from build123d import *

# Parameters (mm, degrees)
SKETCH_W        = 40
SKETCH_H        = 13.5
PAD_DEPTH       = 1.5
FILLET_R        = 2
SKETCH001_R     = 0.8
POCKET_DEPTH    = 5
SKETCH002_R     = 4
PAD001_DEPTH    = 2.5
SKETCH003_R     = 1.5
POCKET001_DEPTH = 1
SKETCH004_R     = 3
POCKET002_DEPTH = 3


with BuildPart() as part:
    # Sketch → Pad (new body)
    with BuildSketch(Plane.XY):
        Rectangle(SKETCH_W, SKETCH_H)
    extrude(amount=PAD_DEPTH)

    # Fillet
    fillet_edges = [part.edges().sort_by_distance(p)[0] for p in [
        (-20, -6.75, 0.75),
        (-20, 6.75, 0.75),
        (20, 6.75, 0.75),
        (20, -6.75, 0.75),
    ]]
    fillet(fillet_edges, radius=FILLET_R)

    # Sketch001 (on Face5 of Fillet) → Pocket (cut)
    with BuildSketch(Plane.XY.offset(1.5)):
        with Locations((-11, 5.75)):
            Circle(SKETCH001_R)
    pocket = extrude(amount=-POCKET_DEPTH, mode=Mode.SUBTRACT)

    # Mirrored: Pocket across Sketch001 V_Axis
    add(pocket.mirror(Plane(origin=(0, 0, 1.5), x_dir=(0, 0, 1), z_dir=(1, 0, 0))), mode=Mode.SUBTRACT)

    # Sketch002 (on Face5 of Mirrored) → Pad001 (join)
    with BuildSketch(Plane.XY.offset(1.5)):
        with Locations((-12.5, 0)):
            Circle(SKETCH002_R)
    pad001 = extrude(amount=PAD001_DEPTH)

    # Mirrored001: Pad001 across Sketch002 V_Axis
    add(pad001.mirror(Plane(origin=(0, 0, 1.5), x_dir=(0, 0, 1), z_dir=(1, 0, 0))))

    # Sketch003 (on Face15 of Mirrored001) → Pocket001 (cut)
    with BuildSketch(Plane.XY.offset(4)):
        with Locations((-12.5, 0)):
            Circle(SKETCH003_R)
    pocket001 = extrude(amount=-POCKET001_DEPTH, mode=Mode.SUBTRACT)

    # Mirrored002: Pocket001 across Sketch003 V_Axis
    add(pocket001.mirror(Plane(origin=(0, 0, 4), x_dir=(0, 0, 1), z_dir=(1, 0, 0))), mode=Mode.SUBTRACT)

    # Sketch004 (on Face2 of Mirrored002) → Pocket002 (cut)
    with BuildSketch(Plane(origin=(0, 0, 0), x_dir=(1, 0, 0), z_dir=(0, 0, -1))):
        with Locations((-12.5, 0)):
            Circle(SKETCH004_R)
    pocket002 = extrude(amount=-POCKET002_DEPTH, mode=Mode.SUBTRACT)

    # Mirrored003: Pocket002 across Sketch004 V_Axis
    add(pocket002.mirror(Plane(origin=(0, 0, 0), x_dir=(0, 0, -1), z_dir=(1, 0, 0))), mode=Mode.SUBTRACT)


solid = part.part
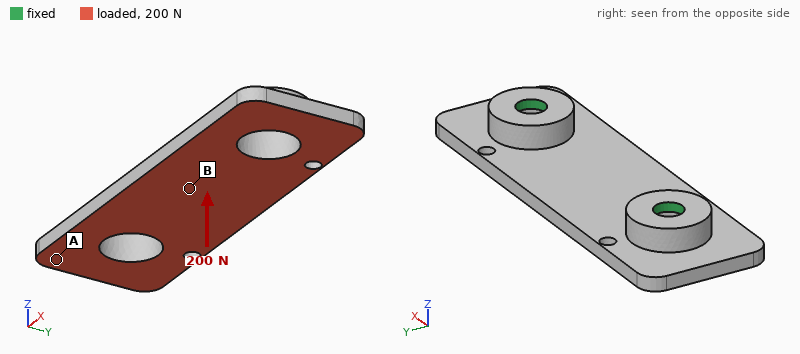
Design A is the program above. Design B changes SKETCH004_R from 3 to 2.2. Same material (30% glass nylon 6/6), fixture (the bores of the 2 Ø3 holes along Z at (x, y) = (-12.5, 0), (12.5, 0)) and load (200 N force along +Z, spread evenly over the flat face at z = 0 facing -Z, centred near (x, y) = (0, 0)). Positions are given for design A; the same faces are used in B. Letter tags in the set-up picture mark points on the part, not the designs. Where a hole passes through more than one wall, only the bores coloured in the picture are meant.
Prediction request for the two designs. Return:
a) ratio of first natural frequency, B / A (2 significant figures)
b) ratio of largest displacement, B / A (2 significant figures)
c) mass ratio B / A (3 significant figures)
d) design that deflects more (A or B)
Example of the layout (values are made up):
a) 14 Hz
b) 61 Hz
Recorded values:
a) 1.1
b) 0.82
c) 1.09
d) A
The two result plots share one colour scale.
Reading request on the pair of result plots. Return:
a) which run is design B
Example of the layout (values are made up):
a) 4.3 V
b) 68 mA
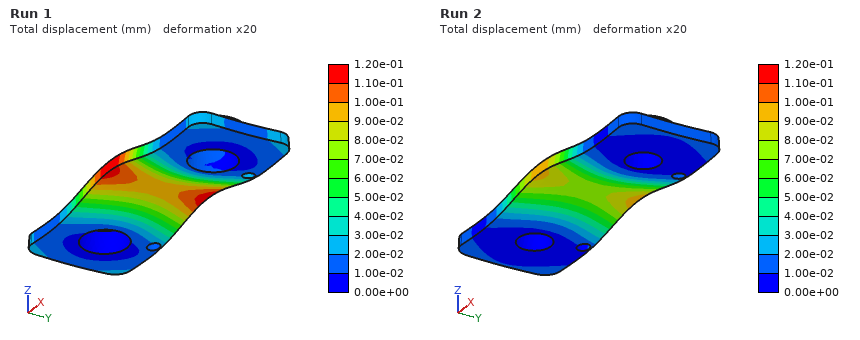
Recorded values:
a) Run 2
